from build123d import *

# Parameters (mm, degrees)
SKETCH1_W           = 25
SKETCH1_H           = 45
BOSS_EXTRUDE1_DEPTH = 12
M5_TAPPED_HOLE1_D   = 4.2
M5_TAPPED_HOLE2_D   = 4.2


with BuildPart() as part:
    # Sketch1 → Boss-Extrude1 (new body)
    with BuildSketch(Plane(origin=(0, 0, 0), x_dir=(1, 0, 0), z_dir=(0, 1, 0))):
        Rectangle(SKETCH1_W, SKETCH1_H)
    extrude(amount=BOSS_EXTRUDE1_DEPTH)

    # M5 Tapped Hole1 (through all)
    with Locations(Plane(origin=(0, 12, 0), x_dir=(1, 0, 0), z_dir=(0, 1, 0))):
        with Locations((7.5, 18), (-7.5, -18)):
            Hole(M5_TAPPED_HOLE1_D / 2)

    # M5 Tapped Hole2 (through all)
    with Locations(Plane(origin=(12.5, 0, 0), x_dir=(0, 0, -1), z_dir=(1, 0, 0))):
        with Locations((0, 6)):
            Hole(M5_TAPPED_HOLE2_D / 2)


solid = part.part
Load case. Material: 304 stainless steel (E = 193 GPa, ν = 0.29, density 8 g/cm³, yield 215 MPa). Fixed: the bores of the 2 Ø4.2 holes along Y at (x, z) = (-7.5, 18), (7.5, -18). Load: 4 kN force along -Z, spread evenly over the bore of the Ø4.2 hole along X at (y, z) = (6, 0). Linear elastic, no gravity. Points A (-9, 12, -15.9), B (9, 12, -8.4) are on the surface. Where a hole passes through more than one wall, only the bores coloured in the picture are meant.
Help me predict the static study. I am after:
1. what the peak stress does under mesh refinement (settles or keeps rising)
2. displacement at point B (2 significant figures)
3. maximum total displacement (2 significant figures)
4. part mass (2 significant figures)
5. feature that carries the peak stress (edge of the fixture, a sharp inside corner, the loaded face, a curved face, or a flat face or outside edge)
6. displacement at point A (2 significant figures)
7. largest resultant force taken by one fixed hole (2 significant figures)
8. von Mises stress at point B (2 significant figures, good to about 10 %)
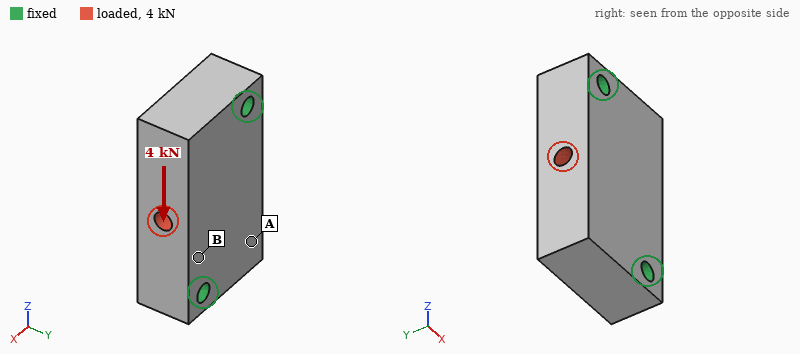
keeps rising
0.77 µm
1.9 µm
100 g
edge of the fixture
1.4 µm
2.0 kN
14 MPa
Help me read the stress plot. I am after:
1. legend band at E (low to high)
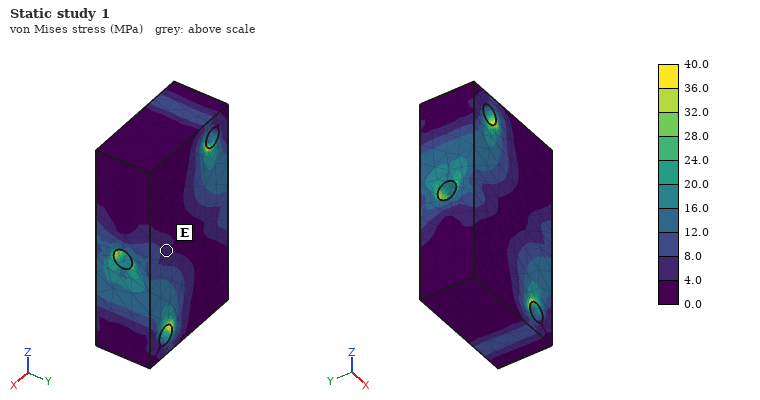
4.0 to 8.0 MPa
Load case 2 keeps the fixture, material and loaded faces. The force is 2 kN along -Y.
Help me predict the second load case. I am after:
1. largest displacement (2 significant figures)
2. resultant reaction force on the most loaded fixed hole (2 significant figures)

2.7 µm
1.0 kN
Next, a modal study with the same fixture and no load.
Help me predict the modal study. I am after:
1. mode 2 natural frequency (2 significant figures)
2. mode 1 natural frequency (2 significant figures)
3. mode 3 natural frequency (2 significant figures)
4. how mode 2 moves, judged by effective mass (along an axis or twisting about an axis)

20 kHz
18 kHz
24 kHz
along Y
